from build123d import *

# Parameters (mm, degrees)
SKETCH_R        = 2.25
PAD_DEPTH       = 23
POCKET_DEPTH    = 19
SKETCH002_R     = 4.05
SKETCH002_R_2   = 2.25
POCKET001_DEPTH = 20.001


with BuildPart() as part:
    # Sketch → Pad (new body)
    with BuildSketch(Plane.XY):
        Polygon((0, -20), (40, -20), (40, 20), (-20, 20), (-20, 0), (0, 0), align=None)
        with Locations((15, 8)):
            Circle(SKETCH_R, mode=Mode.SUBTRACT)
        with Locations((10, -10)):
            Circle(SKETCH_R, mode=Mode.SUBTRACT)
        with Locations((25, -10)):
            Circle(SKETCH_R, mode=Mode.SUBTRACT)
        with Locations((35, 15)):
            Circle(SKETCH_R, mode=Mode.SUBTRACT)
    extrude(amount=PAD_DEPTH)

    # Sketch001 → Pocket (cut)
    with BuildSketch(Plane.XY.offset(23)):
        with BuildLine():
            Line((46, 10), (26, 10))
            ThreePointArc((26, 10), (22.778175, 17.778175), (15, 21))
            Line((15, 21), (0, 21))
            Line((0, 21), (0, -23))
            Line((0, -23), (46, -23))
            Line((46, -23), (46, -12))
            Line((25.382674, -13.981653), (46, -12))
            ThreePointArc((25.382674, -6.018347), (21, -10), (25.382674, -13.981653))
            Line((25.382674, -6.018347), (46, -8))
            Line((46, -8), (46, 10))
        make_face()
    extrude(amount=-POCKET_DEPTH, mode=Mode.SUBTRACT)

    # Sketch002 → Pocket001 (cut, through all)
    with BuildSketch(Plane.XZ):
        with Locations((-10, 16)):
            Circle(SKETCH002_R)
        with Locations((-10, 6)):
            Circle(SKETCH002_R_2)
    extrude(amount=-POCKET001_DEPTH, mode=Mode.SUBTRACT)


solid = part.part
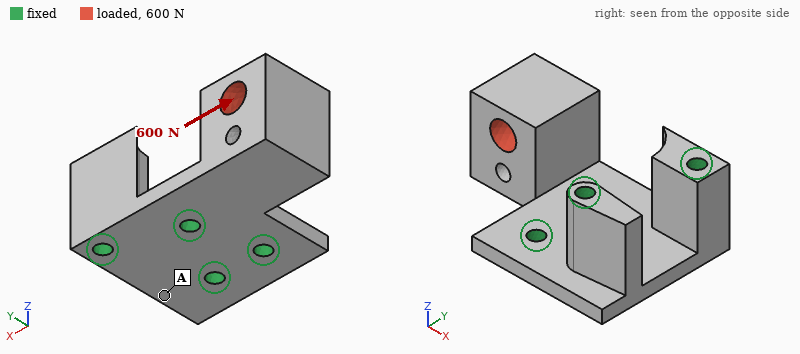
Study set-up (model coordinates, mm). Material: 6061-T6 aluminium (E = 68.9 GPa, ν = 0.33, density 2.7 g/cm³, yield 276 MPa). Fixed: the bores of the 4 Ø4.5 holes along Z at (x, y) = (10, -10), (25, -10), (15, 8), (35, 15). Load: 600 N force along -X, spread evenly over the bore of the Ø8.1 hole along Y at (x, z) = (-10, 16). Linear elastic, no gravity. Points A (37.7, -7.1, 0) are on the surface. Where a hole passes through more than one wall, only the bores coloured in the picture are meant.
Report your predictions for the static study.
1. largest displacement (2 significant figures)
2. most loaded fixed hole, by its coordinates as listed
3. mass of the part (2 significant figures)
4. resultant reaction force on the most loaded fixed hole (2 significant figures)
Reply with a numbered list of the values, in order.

1. 0.47 mm
2. (15, 8)
3. 51 g
4. 480 N
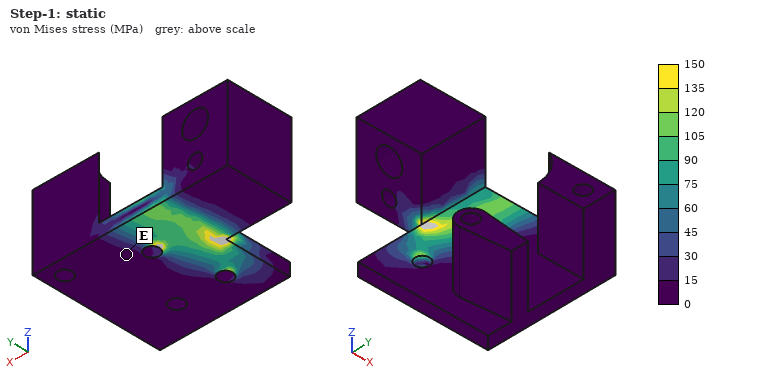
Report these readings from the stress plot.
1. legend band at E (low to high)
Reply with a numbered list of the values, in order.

1. 0 to 15 MPa
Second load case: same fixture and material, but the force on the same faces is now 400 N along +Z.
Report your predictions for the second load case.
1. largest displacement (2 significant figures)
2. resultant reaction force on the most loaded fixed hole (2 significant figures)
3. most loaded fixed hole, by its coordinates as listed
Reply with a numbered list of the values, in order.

1. 0.38 mm
2. 450 N
3. (15, 8)
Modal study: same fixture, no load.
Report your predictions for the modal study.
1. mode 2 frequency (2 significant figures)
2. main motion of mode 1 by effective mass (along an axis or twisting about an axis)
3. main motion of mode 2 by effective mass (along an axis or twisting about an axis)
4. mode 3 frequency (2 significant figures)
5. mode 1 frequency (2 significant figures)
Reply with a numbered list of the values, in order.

1. 3300 Hz
2. along Z
3. along Y
4. 7800 Hz
5. 1300 Hz
